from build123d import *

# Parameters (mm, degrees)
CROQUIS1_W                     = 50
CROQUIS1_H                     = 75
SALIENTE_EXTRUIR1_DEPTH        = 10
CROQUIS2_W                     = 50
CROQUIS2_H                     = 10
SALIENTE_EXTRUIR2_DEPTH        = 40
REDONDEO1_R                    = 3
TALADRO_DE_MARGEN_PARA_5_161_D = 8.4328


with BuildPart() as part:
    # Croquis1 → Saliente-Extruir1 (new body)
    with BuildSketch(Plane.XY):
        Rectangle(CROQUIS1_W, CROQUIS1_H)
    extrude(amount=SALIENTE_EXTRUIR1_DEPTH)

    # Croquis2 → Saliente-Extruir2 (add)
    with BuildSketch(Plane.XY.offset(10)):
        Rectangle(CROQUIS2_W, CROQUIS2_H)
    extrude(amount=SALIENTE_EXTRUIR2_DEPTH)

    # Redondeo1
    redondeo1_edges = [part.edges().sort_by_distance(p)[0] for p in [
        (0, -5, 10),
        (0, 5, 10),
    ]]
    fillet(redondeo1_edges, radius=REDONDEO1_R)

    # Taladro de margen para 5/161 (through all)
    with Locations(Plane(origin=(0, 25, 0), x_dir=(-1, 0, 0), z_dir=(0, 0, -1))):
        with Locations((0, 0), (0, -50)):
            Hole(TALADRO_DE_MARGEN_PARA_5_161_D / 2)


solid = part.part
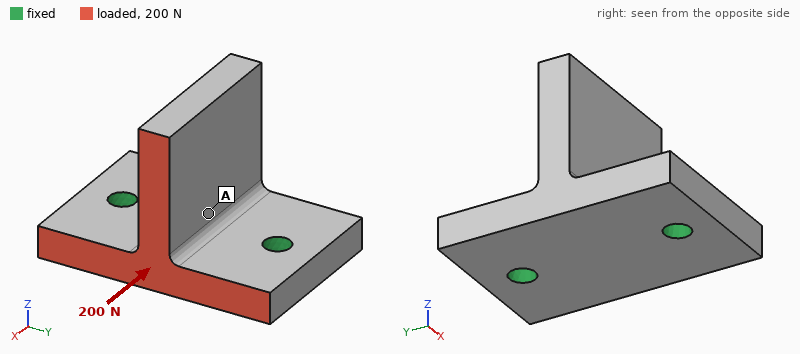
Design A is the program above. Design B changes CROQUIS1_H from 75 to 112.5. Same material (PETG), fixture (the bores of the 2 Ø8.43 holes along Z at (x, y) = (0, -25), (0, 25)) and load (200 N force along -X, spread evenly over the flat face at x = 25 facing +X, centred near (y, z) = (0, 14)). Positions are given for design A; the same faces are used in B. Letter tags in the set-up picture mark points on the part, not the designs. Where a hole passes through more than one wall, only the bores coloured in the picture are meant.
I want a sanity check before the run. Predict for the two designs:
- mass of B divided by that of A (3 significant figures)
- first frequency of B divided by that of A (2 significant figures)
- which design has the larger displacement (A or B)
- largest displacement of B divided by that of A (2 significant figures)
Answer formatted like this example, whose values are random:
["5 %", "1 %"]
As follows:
["1.33", "1.0", "A", "0.70"]
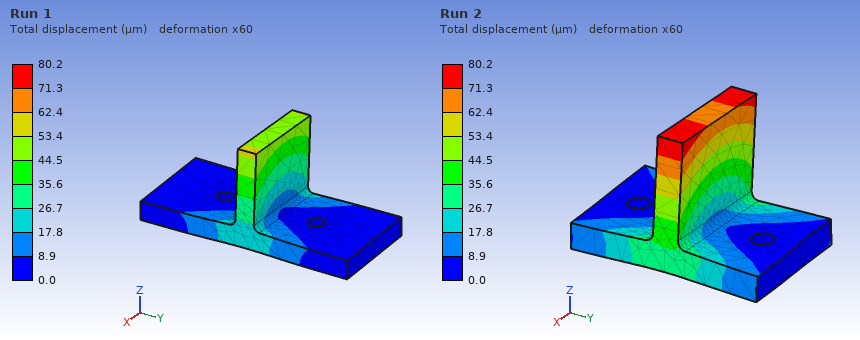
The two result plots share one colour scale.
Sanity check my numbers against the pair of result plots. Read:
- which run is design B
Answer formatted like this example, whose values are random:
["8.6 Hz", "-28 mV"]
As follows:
["Run 1"]
